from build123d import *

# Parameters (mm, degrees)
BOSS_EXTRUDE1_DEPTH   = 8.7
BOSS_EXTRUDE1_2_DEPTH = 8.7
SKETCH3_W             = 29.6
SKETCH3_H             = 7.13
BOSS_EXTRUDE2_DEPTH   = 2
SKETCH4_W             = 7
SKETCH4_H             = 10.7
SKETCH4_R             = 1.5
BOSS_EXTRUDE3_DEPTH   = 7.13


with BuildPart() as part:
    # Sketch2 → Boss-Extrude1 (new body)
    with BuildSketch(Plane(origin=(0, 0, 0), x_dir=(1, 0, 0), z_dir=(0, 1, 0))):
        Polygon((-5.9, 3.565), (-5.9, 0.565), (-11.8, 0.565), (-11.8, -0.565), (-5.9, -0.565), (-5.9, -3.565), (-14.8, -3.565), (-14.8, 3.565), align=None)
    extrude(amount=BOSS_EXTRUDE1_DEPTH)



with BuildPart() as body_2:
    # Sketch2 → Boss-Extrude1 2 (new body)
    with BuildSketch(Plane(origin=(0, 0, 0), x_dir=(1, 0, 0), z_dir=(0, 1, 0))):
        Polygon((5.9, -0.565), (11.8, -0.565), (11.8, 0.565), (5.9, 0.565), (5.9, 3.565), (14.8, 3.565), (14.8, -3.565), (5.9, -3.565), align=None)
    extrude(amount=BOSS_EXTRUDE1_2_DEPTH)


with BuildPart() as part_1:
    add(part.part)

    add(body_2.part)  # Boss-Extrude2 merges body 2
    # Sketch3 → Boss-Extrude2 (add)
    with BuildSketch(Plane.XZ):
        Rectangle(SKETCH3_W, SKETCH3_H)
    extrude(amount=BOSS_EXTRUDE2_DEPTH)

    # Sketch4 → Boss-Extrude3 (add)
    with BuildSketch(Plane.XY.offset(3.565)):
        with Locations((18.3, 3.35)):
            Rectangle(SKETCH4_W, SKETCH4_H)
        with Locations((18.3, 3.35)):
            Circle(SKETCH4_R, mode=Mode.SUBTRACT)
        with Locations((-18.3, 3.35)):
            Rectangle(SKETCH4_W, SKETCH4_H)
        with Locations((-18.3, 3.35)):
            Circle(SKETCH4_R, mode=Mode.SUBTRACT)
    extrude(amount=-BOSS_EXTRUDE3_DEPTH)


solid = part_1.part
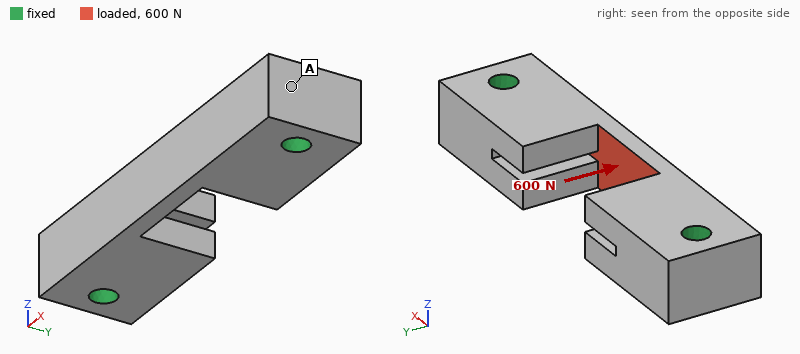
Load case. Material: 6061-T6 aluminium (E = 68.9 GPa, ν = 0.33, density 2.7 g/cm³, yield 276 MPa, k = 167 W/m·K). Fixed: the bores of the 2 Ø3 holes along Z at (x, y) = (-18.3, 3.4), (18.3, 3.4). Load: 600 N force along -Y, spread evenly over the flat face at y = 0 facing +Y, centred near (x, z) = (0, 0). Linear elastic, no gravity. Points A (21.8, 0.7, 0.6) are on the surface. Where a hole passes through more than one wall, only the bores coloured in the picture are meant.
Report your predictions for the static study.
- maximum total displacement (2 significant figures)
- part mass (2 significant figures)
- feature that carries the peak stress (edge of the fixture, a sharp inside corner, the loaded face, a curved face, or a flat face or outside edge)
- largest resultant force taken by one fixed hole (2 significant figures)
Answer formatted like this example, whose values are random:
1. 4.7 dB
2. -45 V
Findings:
1. 27 µm
2. 6.4 g
3. a flat face or outside edge
4. 440 N
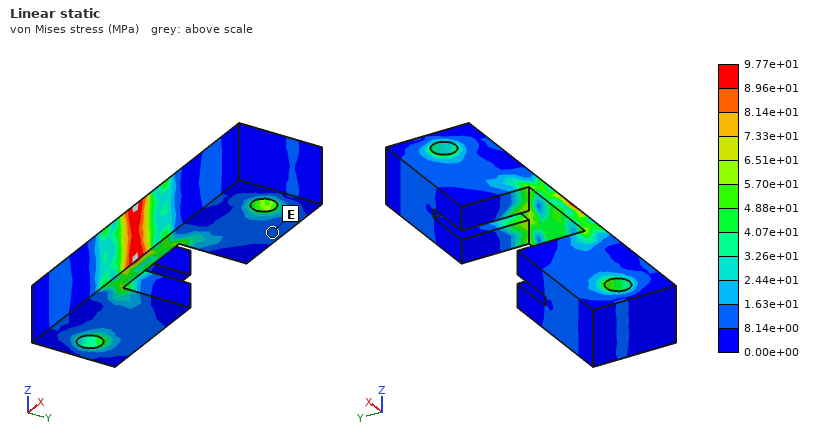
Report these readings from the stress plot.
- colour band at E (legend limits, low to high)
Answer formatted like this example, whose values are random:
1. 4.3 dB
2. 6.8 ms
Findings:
1. 8.14e+00 to 1.63e+01 MPa
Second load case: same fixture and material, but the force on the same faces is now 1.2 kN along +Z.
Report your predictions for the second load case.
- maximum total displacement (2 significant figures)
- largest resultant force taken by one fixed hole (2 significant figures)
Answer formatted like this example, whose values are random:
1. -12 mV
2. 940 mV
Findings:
1. 48 µm
2. 600 N
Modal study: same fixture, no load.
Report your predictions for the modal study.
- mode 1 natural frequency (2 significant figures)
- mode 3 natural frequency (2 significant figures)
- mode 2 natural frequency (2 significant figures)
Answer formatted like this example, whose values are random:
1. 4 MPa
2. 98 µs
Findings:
1. 27 kHz
2. 28 kHz
3. 27 kHz
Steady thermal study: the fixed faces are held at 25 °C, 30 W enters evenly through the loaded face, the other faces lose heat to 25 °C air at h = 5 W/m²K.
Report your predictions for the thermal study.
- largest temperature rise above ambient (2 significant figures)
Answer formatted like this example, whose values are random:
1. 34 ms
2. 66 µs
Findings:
1. 42 K
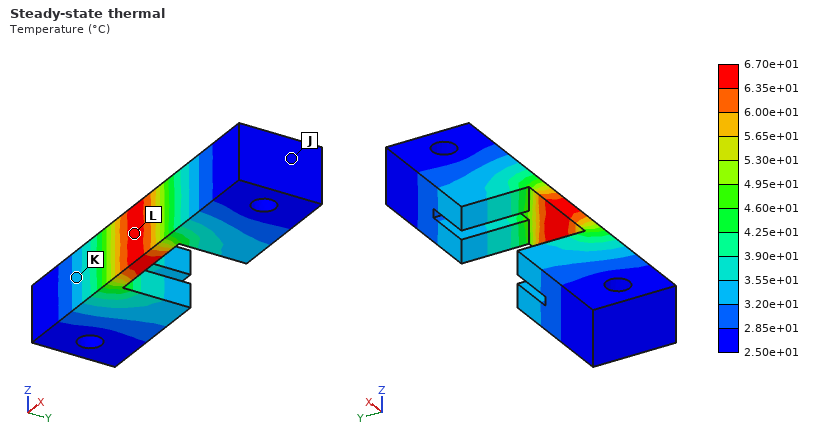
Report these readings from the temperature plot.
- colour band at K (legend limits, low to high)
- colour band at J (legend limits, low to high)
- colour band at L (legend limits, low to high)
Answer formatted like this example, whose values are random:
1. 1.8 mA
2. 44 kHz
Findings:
1. 3.20e+01 to 3.55e+01 °C
2. 2.50e+01 to 2.85e+01 °C
3. 6.35e+01 to 6.70e+01 °C
